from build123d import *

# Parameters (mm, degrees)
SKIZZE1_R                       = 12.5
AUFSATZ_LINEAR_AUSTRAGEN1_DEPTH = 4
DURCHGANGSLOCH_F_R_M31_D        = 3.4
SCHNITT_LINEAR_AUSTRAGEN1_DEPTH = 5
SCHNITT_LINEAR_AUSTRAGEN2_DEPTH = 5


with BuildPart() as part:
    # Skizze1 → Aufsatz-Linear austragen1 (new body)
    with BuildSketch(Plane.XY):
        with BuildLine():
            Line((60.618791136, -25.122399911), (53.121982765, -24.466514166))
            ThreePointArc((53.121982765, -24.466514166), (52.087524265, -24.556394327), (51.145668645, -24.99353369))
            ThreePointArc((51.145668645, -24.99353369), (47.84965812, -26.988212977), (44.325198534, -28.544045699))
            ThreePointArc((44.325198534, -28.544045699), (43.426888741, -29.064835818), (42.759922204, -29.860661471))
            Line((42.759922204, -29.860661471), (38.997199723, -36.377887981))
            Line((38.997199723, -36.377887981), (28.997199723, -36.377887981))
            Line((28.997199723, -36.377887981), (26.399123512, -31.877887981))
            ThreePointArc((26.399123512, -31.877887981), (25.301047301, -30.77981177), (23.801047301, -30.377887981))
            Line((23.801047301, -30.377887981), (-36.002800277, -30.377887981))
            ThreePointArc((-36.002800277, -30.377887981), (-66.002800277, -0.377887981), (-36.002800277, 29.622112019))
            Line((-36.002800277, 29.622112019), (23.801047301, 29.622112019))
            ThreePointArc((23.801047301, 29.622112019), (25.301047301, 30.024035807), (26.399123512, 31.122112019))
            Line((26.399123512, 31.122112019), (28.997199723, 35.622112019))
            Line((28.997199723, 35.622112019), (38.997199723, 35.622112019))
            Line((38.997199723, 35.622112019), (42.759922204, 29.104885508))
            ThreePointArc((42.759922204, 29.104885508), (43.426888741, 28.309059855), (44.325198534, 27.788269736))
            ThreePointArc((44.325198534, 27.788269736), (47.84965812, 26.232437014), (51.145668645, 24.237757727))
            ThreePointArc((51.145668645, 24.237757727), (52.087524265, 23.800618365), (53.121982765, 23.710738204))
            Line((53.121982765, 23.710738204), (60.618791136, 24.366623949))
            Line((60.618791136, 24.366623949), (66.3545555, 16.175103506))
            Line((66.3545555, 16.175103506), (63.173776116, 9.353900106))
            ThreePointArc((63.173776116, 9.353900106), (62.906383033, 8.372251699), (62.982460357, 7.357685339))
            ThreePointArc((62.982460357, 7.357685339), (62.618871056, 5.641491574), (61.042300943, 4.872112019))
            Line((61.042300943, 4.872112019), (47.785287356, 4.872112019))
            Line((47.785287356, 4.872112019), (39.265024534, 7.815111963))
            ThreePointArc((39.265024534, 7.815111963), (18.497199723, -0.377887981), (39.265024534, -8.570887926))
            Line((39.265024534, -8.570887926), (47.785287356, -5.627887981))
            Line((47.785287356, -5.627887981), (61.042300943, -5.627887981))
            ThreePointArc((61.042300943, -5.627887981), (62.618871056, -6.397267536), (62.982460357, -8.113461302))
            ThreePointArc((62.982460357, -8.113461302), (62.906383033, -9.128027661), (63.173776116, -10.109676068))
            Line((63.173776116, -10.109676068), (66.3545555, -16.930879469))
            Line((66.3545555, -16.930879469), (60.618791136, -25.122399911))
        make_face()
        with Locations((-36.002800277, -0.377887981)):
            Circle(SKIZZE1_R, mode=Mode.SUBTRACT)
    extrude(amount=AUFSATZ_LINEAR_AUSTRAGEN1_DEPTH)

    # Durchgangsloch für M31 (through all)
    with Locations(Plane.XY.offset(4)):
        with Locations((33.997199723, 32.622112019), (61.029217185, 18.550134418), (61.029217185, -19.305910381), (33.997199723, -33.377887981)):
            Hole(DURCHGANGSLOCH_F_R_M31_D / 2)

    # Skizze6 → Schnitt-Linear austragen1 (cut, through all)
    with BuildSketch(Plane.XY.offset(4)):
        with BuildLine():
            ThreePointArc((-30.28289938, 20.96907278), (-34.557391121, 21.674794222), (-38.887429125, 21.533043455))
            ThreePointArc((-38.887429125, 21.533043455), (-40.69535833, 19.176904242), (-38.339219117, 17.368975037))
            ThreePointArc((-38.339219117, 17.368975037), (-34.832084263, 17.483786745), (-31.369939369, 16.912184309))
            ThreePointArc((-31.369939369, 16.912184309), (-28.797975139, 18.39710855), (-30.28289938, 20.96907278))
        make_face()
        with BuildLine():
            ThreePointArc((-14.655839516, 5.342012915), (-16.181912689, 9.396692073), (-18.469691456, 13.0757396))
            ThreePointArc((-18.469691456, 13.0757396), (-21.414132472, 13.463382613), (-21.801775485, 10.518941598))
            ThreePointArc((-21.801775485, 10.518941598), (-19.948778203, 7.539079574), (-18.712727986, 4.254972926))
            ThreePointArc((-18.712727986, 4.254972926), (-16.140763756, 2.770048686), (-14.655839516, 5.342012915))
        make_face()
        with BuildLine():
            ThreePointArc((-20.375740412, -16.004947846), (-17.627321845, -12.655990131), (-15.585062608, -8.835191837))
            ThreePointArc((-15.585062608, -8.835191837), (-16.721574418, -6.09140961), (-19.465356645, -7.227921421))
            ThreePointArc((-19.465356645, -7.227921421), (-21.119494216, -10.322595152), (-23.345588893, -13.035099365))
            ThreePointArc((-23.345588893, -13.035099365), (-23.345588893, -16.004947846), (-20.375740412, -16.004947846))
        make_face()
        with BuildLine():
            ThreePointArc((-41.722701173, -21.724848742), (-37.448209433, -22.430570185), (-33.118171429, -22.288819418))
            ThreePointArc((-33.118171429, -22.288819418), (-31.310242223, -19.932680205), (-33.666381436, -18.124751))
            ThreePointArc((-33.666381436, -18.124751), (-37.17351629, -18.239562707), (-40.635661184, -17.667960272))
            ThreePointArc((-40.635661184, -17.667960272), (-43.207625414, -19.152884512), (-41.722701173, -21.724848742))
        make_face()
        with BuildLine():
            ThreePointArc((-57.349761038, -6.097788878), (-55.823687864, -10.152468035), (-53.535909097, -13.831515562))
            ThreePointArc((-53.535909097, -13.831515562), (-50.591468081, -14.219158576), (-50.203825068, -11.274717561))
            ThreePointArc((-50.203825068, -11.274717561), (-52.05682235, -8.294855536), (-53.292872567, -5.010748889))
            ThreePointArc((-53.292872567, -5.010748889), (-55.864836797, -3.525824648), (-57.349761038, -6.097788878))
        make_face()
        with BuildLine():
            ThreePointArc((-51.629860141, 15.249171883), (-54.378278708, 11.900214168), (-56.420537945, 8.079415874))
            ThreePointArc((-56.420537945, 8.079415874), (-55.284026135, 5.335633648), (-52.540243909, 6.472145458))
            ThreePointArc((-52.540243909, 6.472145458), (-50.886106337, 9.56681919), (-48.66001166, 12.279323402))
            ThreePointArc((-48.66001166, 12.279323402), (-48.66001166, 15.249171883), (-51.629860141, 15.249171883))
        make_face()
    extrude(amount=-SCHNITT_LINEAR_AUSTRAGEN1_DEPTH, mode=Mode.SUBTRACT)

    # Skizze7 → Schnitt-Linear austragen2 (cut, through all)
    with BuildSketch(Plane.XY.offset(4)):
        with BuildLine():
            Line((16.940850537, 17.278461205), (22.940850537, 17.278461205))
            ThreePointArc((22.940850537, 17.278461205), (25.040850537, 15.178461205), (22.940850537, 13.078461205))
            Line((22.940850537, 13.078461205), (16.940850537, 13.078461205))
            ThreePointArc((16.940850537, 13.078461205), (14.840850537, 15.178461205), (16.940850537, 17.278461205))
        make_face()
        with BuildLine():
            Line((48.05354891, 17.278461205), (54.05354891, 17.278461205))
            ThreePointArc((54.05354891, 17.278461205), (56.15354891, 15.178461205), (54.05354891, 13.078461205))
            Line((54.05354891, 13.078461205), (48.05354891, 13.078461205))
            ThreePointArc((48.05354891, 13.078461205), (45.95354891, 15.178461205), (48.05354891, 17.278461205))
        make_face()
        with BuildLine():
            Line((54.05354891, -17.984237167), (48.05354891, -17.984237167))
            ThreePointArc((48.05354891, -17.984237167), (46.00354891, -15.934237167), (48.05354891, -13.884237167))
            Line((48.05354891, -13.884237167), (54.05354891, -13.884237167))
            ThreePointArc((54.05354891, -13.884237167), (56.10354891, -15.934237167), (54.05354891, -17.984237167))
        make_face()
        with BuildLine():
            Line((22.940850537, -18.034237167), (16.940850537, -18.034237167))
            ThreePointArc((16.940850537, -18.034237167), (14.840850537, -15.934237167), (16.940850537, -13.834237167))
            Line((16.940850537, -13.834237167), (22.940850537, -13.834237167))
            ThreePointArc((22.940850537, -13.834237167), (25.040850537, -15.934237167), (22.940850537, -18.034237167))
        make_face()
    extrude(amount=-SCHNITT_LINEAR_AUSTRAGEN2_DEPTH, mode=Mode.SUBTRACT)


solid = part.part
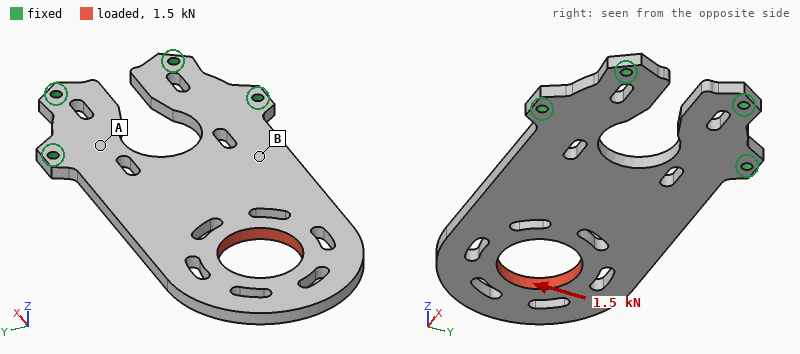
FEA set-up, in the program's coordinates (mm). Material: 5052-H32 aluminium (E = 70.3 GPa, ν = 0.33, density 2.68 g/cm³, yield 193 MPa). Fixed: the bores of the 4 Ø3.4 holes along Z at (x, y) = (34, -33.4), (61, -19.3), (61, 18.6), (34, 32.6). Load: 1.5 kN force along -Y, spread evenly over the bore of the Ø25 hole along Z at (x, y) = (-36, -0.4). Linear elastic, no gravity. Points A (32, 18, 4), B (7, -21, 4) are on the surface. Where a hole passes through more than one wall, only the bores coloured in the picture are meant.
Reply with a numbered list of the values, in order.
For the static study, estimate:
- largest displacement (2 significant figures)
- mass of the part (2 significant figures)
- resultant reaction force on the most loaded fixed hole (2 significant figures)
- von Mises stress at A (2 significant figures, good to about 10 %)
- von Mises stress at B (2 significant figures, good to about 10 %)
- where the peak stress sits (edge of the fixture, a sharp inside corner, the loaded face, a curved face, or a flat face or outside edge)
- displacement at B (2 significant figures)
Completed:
1. 0.11 mm
2. 61 g
3. 1.6 kN
4. 7.8 MPa
5. 22 MPa
6. a curved face
7. 0.022 mm
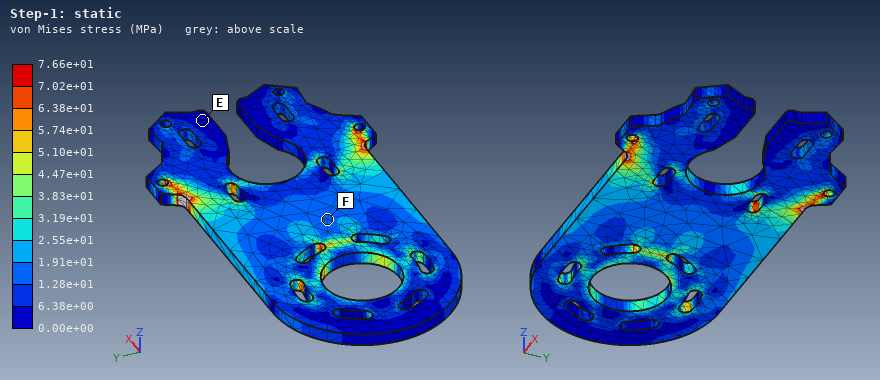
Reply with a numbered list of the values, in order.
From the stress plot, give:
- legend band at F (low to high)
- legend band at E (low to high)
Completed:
1. 1.28e+01 to 1.91e+01 MPa
2. 0.00e+00 to 6.38e+00 MPa
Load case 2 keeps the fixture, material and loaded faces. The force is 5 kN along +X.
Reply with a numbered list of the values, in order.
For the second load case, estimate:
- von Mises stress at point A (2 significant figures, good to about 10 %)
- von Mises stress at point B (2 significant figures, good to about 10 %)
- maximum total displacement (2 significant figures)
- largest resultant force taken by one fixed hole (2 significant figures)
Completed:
1. 17 MPa
2. 29 MPa
3. 58 µm
4. 1.6 kN
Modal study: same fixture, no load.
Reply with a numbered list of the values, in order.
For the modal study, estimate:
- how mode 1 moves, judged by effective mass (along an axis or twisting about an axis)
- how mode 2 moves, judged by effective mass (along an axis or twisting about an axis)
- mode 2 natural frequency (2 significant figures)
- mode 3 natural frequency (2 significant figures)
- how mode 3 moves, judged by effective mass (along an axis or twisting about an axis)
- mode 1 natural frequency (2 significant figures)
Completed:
1. along Z
2. twisting about X
3. 1300 Hz
4. 1800 Hz
5. along Z
6. 330 Hz
